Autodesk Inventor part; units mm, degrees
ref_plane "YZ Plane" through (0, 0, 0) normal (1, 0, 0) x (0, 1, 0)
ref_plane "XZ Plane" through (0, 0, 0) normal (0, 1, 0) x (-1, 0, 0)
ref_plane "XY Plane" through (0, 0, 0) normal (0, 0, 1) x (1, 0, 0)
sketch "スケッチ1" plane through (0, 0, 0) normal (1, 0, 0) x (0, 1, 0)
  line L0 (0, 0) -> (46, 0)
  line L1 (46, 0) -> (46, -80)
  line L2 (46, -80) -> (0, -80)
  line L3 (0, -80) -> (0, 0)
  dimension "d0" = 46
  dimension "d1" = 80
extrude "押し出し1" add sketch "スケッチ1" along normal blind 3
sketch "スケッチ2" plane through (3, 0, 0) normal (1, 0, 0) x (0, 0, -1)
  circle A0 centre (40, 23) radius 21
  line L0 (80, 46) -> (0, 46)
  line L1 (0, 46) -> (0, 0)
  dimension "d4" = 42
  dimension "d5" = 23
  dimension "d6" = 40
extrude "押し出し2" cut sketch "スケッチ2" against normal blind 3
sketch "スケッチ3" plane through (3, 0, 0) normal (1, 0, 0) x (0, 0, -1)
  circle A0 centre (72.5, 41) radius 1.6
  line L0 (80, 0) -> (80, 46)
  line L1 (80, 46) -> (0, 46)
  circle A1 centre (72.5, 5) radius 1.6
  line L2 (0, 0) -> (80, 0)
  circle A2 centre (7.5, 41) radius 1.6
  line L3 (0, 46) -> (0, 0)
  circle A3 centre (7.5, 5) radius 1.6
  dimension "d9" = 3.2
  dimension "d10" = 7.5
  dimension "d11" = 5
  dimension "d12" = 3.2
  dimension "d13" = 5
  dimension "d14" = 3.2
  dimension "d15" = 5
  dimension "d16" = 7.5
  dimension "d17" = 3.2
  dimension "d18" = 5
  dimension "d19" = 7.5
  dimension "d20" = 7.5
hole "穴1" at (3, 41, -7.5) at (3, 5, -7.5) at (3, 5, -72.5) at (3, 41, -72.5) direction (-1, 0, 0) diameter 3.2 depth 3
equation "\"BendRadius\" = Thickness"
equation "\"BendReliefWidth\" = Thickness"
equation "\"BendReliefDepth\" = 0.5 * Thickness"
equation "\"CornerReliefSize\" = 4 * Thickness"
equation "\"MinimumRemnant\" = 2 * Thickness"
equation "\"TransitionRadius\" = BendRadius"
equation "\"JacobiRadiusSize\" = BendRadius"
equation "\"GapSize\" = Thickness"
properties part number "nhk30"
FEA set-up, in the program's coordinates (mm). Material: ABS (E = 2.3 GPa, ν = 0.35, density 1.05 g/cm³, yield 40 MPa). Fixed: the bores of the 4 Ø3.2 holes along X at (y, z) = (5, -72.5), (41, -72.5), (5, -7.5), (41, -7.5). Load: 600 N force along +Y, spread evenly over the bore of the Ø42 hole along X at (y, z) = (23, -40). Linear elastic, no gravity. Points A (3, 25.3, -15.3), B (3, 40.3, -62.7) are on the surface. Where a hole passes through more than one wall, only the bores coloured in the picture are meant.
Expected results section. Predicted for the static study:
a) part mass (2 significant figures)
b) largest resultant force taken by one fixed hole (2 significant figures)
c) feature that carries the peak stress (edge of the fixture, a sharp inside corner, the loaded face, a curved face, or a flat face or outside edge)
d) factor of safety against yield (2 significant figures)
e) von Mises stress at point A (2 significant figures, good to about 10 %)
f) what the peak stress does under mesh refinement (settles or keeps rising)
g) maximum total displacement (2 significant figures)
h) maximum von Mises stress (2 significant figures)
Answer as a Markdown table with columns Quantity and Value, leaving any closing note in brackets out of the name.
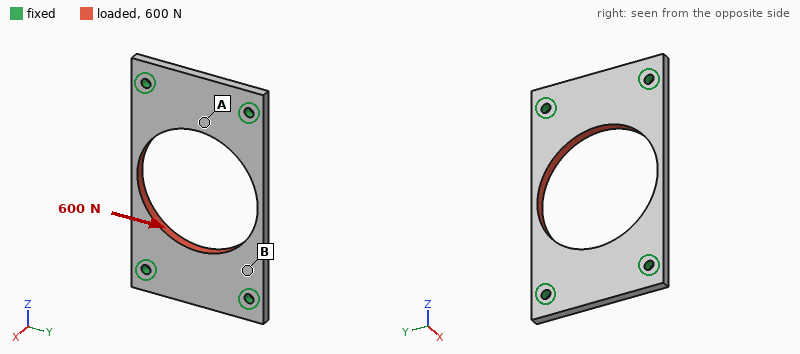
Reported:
| Quantity | Value |
|---|---|
| part mass | 7.1 g |
| largest resultant force taken by one fixed hole | 160 N |
| feature that carries the peak stress | a flat face or outside edge |
| factor of safety against yield | 1.2 |
| von Mises stress at point A | 5.9 MPa |
| what the peak stress does under mesh refinement | settles |
| maximum total displacement | 0.41 mm |
| maximum von Mises stress | 32 MPa |
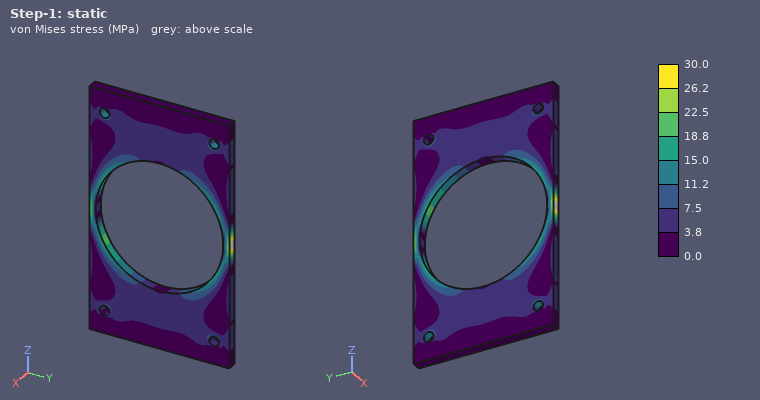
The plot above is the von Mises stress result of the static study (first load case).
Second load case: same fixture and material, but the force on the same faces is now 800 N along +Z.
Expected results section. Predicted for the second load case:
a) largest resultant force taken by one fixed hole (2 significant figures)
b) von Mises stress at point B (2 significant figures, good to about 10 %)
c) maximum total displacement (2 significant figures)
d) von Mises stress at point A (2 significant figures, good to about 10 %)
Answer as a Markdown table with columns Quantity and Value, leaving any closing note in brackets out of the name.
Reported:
| Quantity | Value |
|---|---|
| largest resultant force taken by one fixed hole | 200 N |
| von Mises stress at point B | 4.1 MPa |
| maximum total displacement | 66 µm |
| von Mises stress at point A | 2.1 MPa |
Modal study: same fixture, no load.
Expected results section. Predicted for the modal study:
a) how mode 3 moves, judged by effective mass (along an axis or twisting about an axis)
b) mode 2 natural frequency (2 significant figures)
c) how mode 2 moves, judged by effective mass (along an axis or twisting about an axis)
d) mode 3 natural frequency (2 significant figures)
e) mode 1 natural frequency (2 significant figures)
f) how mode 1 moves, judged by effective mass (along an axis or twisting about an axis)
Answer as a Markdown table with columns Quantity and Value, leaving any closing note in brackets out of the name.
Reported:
| Quantity | Value |
|---|---|
| how mode 3 moves, judged by effective mass | twisting about Y |
| mode 2 natural frequency | 1700 Hz |
| how mode 2 moves, judged by effective mass | twisting about Z |
| mode 3 natural frequency | 2500 Hz |
| mode 1 natural frequency | 1500 Hz |
| how mode 1 moves, judged by effective mass | along X |
